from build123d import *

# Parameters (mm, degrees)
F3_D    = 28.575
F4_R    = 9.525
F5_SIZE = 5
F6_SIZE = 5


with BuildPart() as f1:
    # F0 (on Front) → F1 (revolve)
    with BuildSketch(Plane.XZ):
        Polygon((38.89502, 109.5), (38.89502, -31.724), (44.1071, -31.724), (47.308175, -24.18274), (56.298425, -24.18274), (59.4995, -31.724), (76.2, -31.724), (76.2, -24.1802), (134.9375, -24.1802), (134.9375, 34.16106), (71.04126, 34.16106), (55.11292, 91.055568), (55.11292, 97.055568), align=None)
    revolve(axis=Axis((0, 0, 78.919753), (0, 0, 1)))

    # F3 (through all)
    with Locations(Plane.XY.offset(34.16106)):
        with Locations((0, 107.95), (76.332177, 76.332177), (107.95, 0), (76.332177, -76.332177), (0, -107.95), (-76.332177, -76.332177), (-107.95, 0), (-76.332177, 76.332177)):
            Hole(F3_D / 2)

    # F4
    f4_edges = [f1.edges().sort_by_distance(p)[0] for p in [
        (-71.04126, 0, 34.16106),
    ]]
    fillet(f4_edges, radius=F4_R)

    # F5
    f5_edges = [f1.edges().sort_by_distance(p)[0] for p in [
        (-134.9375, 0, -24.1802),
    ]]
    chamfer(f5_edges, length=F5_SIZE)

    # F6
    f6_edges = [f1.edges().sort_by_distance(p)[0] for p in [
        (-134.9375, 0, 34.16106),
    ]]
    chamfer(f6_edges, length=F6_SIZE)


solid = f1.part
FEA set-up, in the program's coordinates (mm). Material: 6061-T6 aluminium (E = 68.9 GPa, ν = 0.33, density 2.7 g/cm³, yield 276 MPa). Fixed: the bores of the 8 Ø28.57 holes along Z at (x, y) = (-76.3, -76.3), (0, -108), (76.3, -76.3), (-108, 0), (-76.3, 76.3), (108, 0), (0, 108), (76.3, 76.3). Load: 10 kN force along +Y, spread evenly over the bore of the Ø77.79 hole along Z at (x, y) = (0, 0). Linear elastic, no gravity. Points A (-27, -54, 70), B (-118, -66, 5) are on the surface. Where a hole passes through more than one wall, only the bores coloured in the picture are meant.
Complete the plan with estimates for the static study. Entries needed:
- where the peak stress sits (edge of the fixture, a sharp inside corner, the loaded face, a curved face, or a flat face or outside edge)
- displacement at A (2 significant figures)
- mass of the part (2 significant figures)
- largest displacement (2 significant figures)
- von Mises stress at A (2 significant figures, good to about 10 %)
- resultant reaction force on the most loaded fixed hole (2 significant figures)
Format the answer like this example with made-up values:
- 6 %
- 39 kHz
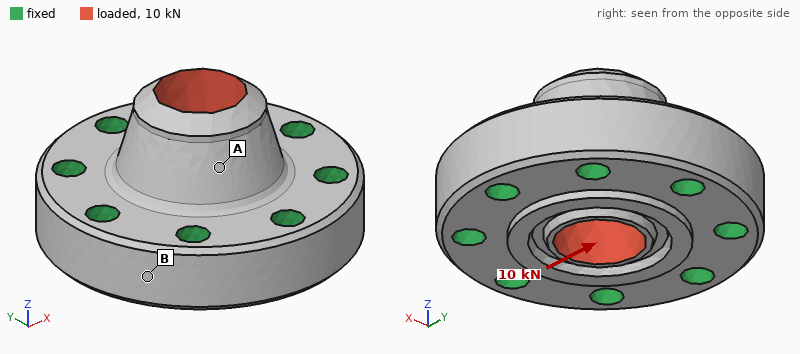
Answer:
- a curved face
- 1.8 µm
- 9.0 kg
- 3.8 µm
- 0.76 MPa
- 2.2 kN
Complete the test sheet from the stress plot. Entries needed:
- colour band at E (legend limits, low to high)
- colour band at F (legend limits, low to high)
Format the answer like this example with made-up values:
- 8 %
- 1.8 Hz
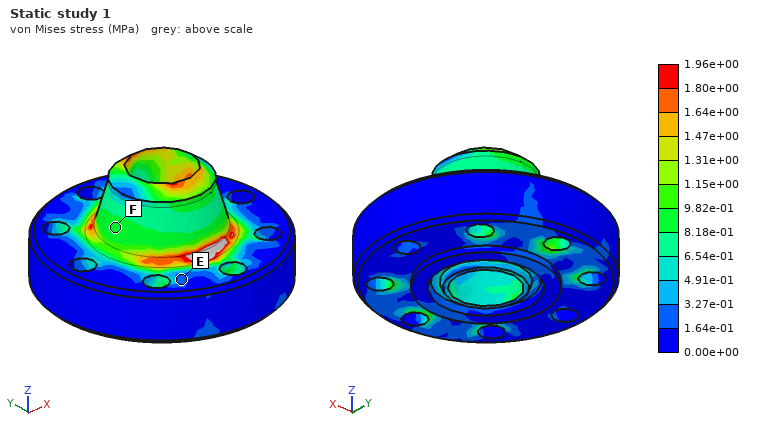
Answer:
- 1.64e-01 to 3.27e-01 MPa
- 8.18e-01 to 9.82e-01 MPa
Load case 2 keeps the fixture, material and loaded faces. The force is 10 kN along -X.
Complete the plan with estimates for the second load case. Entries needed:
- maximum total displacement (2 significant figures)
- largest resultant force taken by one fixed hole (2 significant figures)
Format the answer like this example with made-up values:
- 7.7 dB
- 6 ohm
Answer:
- 3.9 µm
- 2.2 kN
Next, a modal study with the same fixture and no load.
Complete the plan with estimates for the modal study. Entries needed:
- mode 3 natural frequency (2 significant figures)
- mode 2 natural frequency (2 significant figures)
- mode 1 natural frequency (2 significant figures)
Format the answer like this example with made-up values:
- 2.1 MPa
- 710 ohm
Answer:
- 8600 Hz
- 8100 Hz
- 8100 Hz
